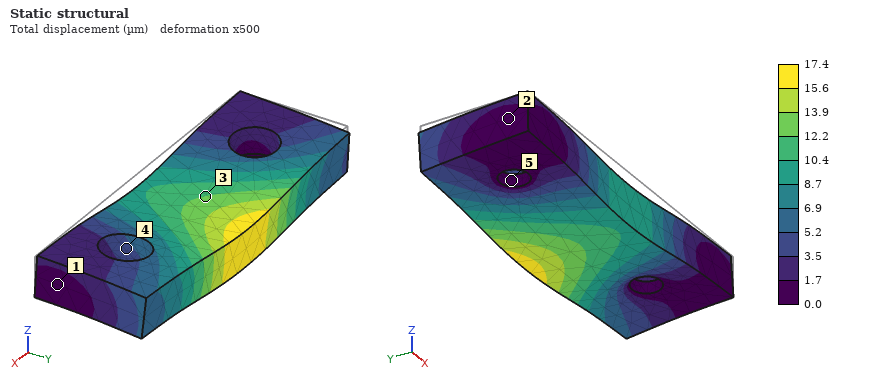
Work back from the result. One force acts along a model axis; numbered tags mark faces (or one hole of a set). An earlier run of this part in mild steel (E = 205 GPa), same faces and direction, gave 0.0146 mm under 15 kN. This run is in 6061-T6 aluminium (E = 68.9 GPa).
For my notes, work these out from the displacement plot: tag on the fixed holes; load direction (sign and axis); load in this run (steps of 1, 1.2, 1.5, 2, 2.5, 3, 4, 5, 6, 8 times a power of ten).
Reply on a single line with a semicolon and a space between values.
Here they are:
5; -Z; 6 kN
